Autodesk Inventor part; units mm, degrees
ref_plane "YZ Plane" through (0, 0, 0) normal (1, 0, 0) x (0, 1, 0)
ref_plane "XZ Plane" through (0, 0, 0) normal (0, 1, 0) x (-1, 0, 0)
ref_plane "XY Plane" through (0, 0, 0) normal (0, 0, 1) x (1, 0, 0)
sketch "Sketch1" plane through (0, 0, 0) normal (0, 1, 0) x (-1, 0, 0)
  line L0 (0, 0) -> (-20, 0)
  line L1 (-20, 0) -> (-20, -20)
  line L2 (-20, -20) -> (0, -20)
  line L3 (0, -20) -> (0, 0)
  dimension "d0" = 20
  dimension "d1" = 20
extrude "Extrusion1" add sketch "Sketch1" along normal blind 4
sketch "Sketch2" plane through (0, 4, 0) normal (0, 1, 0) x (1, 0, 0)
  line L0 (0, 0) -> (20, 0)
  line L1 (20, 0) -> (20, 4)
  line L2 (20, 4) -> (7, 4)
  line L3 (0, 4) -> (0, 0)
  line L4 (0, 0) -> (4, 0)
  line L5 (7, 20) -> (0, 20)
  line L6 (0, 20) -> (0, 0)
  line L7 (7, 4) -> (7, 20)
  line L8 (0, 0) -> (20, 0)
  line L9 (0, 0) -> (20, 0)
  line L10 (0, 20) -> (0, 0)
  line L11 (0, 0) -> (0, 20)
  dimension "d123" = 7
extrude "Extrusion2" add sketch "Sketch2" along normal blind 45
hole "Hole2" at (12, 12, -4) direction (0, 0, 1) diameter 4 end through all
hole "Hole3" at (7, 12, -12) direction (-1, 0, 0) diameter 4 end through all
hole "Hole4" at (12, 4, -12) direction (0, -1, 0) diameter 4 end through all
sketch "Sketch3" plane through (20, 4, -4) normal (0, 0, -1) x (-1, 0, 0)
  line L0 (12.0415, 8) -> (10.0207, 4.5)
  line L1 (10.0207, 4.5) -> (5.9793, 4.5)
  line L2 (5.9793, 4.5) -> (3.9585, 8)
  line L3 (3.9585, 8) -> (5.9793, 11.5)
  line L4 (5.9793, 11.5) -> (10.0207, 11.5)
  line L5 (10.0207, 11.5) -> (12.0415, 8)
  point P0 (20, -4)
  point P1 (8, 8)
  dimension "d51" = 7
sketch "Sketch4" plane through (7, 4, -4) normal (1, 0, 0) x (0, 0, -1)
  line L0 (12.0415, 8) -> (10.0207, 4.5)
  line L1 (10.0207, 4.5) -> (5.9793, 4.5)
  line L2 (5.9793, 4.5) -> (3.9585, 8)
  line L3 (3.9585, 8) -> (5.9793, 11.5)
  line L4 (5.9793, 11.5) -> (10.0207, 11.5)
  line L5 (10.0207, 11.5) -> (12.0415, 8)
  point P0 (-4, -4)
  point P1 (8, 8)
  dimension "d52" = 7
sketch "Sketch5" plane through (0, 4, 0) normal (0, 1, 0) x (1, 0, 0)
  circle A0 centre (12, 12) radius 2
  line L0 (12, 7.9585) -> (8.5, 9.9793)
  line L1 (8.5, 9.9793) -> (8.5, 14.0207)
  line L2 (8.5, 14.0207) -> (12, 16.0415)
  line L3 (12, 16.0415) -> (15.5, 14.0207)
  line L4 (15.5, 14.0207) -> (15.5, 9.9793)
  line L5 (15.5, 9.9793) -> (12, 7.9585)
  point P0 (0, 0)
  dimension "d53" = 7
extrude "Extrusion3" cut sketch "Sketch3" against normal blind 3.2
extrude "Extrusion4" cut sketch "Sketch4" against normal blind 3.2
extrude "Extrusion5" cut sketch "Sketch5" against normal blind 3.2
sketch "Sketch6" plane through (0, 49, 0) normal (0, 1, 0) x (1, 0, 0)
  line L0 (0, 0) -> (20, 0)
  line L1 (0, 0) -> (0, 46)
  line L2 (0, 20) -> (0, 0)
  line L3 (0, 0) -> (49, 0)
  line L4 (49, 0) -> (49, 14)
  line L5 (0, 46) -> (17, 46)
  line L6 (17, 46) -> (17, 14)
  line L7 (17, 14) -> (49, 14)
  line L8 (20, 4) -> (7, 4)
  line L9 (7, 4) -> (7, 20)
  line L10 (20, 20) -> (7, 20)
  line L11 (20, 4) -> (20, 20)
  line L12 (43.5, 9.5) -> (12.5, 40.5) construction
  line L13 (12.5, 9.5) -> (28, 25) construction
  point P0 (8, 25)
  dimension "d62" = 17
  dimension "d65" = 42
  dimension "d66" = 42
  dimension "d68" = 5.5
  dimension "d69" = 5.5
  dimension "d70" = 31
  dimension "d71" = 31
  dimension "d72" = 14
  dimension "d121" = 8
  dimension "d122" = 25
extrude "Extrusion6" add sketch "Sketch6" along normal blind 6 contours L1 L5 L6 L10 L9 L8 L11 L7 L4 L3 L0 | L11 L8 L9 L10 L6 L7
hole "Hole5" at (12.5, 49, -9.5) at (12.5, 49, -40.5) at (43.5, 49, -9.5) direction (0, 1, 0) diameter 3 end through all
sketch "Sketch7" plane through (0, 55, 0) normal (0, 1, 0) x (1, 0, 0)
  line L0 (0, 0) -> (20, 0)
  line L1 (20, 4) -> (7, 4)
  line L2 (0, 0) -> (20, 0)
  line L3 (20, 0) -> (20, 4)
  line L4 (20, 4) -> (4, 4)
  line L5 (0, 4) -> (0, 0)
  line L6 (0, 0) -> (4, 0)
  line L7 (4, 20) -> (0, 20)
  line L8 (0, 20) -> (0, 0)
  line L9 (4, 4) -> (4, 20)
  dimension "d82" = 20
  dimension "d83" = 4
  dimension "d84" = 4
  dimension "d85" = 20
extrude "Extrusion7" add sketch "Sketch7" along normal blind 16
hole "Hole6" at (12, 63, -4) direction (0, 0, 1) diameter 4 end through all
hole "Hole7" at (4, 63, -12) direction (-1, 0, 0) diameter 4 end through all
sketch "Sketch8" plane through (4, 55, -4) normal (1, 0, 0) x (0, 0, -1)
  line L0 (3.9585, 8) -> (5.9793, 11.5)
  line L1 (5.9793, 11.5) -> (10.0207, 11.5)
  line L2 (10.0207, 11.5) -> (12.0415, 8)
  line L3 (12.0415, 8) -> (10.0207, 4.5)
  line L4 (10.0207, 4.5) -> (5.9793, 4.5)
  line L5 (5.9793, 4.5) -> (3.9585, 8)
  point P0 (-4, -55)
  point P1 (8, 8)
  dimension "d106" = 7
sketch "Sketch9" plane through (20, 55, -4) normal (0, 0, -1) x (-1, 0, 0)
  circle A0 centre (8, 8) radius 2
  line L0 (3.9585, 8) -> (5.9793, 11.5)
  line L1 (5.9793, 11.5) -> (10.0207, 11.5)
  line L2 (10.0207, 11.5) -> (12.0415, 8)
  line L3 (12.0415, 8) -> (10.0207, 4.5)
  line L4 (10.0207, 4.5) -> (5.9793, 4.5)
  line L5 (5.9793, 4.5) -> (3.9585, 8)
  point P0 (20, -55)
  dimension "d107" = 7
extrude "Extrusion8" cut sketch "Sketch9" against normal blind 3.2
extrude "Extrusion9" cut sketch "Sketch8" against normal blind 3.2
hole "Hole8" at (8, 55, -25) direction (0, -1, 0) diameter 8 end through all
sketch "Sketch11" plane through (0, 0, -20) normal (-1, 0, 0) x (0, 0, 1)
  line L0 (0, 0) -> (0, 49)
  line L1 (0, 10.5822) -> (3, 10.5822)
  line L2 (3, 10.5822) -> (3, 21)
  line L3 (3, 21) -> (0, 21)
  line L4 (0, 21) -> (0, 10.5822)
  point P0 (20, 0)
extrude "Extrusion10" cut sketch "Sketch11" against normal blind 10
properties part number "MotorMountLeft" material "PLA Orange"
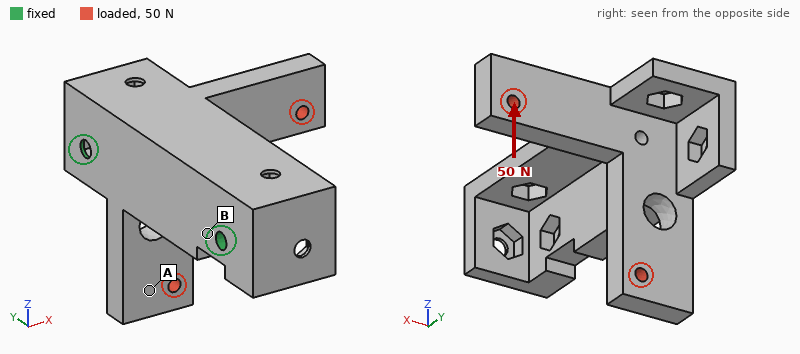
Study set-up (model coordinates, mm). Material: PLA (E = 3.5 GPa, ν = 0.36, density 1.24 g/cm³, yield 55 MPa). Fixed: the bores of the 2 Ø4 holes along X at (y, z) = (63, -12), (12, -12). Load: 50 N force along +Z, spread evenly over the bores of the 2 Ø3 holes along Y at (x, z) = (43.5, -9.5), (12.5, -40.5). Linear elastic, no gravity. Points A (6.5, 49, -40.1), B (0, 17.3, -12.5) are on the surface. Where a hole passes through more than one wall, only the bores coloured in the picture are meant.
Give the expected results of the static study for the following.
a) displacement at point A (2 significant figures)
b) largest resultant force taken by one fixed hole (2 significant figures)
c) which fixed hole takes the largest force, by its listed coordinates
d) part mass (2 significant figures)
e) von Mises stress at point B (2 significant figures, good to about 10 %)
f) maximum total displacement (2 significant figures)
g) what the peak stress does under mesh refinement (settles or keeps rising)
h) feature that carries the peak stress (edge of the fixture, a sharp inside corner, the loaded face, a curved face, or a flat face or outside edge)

0.59 mm
41 N
(63, -12)
23 g
8.4 MPa
1.1 mm
keeps rising
edge of the fixture
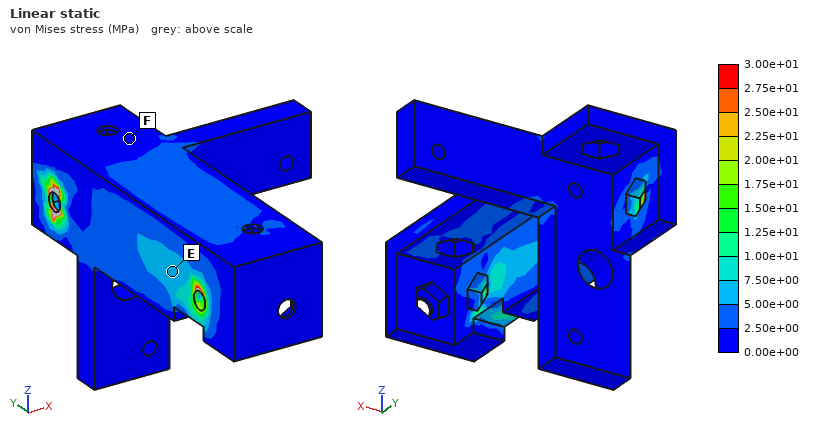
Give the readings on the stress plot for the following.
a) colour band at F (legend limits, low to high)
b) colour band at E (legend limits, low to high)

0.00e+00 to 2.50e+00 MPa
5.00e+00 to 7.50e+00 MPa
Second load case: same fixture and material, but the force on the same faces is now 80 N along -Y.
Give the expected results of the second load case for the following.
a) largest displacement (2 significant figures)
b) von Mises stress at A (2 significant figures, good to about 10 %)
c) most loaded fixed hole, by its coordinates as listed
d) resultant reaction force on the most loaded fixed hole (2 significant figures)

0.68 mm
1.3 MPa
(12, -12)
82 N
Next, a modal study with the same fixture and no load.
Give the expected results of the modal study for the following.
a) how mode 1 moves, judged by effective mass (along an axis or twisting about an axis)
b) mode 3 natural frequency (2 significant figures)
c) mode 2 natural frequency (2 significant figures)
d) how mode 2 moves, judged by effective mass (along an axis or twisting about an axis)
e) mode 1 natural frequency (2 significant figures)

along Z
1400 Hz
1200 Hz
along Y
500 Hz
